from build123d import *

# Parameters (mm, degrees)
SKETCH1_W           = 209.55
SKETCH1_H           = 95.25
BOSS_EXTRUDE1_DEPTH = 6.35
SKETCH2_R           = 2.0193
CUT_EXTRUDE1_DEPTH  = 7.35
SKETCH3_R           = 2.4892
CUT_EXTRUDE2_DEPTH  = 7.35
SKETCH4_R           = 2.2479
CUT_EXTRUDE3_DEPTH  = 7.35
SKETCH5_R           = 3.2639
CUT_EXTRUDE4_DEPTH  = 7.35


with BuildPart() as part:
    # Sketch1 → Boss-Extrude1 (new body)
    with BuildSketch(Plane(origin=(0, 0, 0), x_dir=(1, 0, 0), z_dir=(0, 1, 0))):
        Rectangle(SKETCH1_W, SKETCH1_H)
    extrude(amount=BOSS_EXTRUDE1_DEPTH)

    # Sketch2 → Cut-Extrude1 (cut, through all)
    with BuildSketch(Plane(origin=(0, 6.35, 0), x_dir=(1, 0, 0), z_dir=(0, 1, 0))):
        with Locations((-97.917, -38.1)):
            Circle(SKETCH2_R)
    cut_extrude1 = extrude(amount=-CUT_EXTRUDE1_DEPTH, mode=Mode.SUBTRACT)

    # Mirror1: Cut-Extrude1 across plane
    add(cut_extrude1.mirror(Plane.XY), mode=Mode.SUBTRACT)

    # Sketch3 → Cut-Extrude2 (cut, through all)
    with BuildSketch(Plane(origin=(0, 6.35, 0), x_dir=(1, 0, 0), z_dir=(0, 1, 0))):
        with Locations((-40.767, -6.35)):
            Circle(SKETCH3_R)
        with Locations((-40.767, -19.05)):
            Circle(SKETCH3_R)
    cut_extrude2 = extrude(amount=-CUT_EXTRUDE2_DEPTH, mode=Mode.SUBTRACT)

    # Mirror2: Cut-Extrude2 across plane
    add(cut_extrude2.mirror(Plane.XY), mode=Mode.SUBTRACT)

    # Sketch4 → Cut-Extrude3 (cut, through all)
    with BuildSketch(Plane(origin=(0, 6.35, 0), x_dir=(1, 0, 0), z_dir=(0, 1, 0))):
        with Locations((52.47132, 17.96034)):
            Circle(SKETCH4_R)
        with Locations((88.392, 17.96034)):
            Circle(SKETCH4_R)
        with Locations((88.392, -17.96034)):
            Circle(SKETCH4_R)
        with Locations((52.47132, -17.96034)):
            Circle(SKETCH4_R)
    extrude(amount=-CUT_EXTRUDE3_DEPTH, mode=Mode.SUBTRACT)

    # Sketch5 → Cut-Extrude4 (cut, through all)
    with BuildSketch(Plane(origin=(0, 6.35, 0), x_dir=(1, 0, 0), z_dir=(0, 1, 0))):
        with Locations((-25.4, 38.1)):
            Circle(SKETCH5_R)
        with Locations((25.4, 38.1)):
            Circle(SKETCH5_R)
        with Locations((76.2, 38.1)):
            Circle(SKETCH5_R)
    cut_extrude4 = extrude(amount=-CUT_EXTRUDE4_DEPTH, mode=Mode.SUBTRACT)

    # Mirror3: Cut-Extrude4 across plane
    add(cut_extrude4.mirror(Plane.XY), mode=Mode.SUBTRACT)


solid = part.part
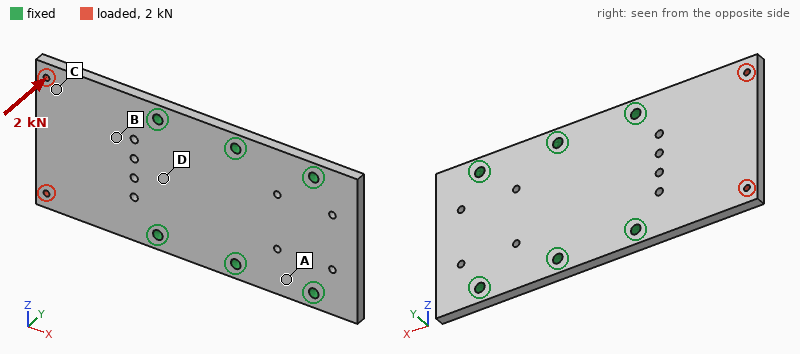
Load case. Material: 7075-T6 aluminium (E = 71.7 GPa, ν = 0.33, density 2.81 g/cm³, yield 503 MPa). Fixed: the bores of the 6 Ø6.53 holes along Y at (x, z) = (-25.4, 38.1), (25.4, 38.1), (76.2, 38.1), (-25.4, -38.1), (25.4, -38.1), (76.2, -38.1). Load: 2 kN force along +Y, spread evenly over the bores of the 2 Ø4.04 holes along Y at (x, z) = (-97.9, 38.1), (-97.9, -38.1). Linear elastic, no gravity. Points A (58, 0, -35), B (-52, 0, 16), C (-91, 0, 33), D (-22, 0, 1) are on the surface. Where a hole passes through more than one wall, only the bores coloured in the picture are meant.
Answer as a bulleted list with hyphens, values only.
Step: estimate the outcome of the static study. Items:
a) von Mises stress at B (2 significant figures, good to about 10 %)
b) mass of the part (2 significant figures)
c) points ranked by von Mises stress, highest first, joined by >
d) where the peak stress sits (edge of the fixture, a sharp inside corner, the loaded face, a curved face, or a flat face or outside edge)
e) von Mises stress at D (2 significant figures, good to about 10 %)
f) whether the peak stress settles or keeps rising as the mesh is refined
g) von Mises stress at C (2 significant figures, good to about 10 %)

- 120 MPa
- 350 g
- B > D > C > A
- edge of the fixture
- 92 MPa
- keeps rising
- 49 MPa
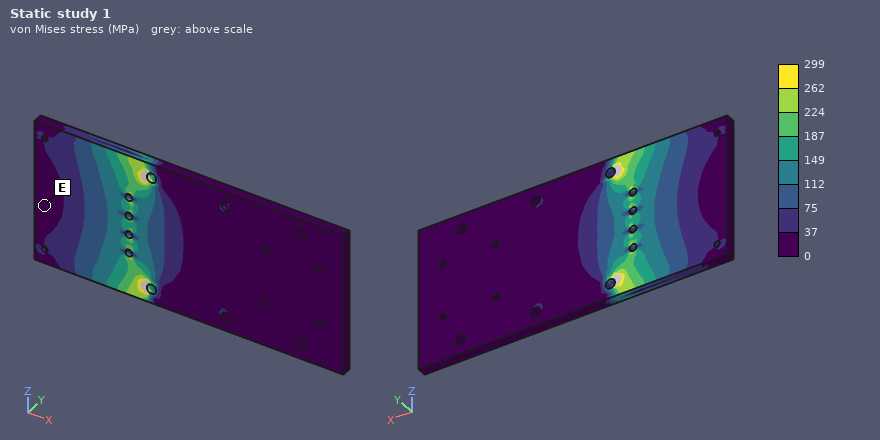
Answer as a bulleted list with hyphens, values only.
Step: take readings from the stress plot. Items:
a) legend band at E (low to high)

- 0 to 37 MPa
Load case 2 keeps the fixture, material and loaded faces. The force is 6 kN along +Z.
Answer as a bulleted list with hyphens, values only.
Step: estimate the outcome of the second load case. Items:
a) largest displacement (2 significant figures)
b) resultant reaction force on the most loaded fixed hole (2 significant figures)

- 76 µm
- 5.9 kN
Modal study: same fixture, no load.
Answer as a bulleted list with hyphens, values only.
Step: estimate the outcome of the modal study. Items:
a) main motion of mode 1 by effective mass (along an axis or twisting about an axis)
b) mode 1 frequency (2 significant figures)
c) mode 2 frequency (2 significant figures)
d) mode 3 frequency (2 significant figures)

- along Y
- 750 Hz
- 1800 Hz
- 4100 Hz
